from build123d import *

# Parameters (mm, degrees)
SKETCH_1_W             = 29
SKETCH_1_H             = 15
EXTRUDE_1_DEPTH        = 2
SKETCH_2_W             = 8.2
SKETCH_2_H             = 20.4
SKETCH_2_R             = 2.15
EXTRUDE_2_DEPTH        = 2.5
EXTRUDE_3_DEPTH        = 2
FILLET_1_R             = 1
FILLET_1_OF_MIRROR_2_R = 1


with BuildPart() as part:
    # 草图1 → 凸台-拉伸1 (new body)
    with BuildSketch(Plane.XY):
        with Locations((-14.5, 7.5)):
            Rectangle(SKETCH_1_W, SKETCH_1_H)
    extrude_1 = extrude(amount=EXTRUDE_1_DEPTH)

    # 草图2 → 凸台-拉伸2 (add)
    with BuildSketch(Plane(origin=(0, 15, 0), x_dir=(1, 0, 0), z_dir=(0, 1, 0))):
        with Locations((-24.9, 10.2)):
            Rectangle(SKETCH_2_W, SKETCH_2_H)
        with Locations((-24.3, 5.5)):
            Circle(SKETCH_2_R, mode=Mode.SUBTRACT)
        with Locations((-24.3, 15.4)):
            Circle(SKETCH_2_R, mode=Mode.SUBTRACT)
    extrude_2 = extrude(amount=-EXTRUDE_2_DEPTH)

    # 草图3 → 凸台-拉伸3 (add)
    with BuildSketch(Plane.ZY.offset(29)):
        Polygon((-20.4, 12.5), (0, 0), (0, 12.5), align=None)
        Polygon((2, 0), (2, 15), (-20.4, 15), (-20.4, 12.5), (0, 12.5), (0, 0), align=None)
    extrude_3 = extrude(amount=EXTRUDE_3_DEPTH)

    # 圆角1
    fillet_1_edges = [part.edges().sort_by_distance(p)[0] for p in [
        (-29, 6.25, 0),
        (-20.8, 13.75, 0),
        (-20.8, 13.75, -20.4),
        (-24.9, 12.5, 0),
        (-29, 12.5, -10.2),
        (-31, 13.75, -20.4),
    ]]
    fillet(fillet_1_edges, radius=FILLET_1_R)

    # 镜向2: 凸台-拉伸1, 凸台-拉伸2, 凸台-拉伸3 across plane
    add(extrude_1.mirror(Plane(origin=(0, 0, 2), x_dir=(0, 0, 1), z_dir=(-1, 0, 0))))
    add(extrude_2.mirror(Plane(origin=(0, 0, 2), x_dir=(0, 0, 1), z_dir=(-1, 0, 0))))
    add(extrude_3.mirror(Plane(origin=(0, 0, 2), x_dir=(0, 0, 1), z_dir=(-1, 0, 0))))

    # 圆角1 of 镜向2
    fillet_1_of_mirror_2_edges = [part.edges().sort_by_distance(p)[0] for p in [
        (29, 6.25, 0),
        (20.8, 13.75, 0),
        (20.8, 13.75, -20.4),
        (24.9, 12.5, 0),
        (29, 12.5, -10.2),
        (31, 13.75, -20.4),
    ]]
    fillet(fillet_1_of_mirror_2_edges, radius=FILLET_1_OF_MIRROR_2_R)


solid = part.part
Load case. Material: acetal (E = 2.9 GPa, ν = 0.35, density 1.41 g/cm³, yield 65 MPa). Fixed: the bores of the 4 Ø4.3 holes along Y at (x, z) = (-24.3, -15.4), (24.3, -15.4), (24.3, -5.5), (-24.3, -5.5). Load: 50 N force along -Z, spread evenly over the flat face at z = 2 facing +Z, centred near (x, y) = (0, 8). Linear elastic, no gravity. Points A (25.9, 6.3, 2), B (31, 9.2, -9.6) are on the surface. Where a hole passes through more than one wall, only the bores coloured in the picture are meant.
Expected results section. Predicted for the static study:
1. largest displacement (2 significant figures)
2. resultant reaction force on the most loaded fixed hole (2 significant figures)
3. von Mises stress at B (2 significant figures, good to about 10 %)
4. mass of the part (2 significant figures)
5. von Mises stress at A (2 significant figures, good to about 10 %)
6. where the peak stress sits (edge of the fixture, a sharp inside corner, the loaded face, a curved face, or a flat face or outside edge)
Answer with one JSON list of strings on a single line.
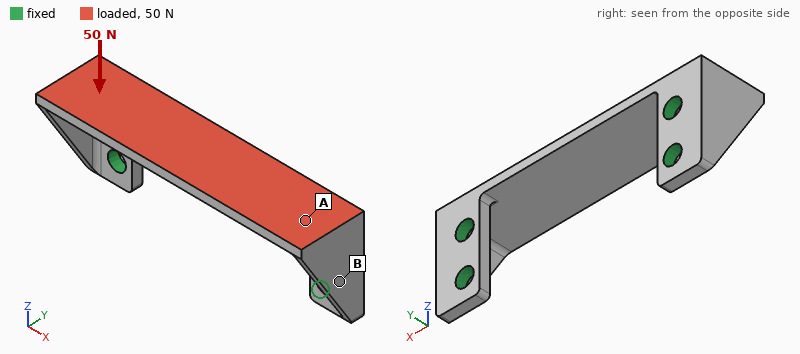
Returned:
["0.69 mm", "28 N", "2.1 MPa", "4.6 g", "7.5 MPa", "a curved face"]
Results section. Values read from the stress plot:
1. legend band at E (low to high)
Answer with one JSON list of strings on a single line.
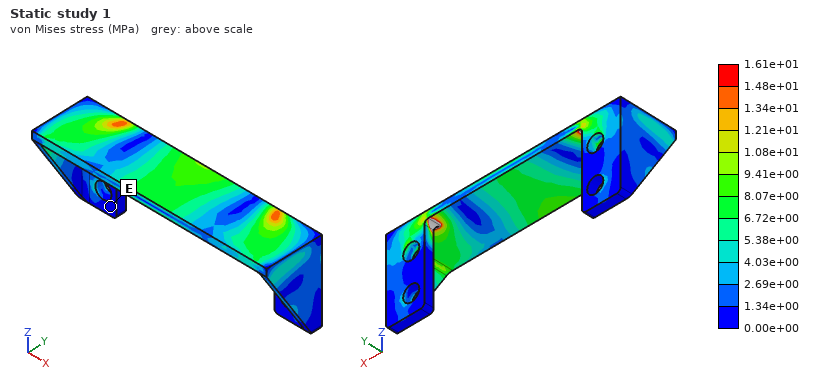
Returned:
["0.00e+00 to 1.34e+00 MPa"]
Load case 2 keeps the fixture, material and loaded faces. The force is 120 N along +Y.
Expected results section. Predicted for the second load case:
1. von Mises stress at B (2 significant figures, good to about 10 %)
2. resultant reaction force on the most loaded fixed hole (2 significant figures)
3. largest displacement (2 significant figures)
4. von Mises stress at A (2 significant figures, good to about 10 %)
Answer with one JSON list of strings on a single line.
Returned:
["3.0 MPa", "79 N", "0.37 mm", "3.8 MPa"]
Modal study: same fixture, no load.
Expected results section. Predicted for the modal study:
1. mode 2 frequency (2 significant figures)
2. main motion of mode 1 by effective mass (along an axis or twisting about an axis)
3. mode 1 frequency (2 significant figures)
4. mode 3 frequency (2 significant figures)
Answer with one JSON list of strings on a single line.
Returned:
["2500 Hz", "along Z", "1100 Hz", "2600 Hz"]
